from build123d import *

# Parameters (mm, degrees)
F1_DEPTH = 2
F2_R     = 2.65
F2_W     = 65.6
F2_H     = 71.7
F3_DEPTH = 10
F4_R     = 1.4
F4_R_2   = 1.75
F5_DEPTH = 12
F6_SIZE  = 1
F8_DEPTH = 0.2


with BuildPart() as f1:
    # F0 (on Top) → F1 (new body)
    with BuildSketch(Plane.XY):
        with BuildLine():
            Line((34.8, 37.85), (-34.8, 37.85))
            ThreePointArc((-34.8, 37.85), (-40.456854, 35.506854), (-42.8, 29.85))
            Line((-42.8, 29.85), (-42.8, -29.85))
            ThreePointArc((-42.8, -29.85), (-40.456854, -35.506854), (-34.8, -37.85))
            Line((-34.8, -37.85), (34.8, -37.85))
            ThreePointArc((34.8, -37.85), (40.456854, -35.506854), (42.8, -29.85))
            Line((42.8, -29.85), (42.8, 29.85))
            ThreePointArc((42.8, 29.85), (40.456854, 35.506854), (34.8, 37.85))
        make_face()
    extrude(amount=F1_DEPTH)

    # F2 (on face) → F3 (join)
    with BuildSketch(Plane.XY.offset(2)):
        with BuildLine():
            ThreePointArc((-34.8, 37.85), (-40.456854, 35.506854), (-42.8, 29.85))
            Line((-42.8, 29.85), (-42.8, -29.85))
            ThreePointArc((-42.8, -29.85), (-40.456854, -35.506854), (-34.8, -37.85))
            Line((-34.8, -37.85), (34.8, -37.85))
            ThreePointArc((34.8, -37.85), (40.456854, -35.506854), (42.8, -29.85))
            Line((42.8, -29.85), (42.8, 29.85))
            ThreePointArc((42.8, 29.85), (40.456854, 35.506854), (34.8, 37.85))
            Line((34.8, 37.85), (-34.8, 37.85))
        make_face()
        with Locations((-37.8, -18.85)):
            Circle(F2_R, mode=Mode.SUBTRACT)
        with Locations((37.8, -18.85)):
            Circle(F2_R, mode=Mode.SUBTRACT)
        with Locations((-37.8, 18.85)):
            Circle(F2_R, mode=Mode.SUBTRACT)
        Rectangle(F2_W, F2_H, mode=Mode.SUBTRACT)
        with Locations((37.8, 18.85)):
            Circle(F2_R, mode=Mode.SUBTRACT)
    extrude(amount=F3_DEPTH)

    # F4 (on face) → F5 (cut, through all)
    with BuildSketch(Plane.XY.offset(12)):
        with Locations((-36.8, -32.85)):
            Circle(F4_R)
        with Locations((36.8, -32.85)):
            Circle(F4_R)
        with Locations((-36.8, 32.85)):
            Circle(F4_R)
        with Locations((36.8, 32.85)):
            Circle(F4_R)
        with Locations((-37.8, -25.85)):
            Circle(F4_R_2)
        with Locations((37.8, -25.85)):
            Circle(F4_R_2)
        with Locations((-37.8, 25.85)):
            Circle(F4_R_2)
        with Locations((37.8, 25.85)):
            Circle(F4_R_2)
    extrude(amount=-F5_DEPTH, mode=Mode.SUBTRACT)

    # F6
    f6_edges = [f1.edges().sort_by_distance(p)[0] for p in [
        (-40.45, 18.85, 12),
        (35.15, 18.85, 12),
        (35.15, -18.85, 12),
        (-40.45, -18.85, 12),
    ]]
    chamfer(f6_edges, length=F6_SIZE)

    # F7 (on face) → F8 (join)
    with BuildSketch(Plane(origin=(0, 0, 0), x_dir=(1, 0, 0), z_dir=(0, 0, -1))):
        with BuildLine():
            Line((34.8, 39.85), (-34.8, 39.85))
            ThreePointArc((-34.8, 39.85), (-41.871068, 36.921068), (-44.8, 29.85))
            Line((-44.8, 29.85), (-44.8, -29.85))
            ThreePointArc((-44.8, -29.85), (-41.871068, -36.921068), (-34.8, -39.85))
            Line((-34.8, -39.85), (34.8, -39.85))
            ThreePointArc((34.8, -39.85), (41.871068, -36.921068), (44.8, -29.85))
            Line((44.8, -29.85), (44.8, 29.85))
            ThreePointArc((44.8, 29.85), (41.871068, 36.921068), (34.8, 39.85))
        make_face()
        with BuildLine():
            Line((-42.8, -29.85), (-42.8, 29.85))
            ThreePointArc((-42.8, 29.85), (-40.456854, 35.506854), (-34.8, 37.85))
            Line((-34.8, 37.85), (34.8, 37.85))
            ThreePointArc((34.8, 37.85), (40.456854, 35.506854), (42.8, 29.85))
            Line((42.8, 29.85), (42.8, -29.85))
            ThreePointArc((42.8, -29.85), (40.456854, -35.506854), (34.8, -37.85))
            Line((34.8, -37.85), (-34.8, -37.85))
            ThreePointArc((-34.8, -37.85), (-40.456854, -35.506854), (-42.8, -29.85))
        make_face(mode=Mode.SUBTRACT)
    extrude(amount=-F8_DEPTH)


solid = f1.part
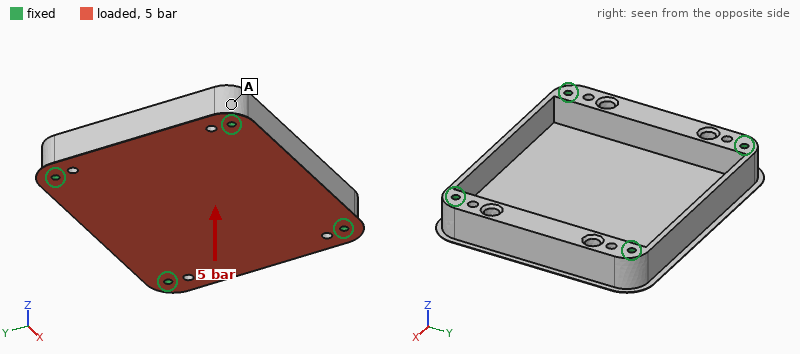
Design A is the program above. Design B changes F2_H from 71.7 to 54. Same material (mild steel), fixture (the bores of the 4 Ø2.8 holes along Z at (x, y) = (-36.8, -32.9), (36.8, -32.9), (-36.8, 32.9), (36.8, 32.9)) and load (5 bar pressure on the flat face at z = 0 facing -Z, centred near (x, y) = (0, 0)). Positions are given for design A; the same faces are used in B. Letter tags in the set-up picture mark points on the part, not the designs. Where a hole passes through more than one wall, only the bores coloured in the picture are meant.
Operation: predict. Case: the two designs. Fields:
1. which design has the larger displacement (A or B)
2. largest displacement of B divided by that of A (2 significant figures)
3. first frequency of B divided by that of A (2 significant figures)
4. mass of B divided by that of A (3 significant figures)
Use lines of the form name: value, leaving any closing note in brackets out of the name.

which design has the larger displacement: A
largest displacement of B divided by that of A: 0.44
first frequency of B divided by that of A: 1.5
mass of B divided by that of A: 1.41
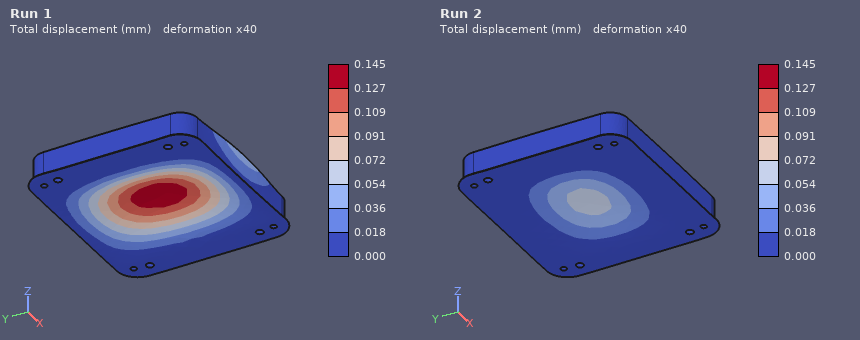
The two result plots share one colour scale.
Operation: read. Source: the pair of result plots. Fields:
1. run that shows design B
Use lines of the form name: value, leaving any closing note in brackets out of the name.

run that shows design B: Run 2
